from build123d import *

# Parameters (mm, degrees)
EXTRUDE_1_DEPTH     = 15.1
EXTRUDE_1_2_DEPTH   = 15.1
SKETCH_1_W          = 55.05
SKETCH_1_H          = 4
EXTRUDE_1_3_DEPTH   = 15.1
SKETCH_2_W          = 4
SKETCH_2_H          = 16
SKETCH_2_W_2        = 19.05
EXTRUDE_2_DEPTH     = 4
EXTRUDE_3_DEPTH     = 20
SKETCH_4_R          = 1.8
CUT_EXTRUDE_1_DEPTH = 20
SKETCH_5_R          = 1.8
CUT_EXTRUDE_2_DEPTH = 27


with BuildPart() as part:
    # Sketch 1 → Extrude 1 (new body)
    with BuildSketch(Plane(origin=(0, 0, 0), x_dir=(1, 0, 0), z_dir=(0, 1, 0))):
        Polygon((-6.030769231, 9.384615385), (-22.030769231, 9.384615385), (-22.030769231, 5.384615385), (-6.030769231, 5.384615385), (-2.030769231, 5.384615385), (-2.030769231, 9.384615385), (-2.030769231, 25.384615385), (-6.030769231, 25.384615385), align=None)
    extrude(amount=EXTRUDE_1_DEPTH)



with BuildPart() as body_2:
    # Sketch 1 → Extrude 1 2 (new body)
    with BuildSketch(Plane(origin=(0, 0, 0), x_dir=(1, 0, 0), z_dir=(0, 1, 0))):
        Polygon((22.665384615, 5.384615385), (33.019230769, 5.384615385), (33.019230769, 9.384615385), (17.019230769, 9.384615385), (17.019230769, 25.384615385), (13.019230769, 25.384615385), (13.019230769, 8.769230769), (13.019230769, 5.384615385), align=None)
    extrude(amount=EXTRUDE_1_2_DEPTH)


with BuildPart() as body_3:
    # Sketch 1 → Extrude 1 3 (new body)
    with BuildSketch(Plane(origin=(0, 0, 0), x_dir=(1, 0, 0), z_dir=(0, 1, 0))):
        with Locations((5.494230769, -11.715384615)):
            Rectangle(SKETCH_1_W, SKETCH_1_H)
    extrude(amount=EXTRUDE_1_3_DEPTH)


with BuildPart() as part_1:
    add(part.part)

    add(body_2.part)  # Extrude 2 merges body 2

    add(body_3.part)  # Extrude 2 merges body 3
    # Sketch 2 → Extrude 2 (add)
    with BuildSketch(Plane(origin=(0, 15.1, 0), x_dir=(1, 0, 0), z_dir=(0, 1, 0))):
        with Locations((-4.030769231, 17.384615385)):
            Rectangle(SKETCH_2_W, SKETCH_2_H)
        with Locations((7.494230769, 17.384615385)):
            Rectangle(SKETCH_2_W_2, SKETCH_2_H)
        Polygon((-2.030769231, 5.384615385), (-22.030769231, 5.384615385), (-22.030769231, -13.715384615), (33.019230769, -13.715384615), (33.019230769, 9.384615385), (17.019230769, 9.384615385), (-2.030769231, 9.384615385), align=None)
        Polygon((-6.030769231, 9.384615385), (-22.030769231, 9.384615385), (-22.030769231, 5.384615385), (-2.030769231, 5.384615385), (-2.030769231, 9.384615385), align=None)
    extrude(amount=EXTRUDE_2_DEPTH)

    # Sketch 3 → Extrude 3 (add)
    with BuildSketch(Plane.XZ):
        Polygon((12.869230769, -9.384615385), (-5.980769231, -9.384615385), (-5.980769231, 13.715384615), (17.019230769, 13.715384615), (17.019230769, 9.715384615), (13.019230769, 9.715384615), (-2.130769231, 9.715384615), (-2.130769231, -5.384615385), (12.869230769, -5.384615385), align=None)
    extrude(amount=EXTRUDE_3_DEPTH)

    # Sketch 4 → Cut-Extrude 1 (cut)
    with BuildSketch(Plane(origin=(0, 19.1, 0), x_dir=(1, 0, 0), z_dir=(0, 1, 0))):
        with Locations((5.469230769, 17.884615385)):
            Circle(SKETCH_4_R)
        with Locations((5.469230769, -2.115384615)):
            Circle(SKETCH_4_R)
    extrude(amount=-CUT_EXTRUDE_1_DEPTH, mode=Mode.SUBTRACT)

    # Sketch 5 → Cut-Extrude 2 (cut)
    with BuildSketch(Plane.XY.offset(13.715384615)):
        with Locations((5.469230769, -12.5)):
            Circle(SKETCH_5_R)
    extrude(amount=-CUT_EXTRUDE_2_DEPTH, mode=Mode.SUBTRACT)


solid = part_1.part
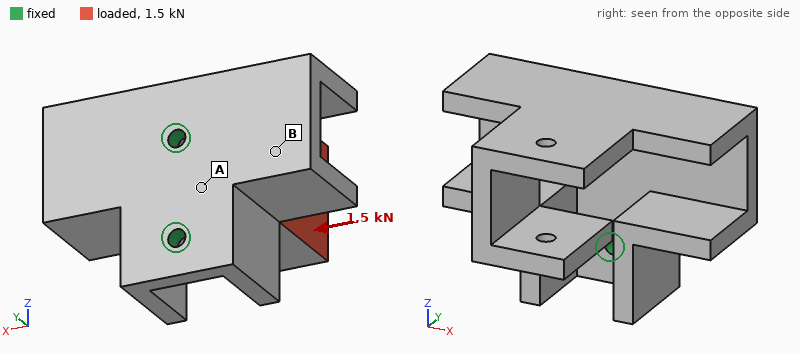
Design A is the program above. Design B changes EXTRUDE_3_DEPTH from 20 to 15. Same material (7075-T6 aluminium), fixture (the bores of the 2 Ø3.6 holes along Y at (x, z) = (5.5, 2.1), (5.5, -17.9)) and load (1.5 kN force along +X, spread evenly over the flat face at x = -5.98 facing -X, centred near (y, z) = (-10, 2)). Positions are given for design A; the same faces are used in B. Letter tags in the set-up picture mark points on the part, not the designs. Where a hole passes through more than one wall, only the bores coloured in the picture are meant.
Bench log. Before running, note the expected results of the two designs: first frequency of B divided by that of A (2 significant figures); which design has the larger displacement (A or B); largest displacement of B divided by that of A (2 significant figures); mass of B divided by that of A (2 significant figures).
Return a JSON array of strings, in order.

["1.1", "A", "0.82", "0.94"]
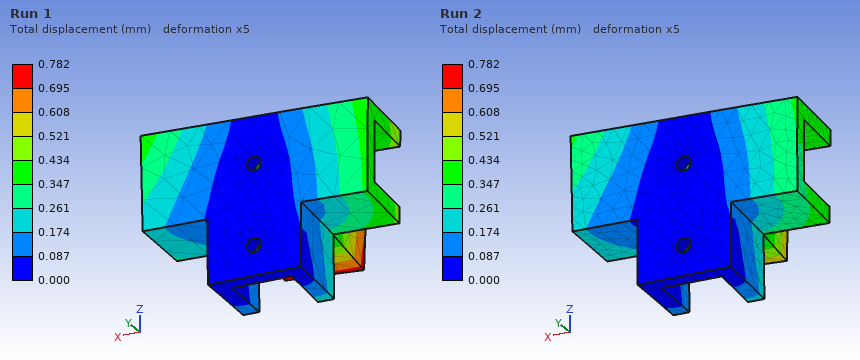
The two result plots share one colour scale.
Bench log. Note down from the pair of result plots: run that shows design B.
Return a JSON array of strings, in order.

["Run 2"]
